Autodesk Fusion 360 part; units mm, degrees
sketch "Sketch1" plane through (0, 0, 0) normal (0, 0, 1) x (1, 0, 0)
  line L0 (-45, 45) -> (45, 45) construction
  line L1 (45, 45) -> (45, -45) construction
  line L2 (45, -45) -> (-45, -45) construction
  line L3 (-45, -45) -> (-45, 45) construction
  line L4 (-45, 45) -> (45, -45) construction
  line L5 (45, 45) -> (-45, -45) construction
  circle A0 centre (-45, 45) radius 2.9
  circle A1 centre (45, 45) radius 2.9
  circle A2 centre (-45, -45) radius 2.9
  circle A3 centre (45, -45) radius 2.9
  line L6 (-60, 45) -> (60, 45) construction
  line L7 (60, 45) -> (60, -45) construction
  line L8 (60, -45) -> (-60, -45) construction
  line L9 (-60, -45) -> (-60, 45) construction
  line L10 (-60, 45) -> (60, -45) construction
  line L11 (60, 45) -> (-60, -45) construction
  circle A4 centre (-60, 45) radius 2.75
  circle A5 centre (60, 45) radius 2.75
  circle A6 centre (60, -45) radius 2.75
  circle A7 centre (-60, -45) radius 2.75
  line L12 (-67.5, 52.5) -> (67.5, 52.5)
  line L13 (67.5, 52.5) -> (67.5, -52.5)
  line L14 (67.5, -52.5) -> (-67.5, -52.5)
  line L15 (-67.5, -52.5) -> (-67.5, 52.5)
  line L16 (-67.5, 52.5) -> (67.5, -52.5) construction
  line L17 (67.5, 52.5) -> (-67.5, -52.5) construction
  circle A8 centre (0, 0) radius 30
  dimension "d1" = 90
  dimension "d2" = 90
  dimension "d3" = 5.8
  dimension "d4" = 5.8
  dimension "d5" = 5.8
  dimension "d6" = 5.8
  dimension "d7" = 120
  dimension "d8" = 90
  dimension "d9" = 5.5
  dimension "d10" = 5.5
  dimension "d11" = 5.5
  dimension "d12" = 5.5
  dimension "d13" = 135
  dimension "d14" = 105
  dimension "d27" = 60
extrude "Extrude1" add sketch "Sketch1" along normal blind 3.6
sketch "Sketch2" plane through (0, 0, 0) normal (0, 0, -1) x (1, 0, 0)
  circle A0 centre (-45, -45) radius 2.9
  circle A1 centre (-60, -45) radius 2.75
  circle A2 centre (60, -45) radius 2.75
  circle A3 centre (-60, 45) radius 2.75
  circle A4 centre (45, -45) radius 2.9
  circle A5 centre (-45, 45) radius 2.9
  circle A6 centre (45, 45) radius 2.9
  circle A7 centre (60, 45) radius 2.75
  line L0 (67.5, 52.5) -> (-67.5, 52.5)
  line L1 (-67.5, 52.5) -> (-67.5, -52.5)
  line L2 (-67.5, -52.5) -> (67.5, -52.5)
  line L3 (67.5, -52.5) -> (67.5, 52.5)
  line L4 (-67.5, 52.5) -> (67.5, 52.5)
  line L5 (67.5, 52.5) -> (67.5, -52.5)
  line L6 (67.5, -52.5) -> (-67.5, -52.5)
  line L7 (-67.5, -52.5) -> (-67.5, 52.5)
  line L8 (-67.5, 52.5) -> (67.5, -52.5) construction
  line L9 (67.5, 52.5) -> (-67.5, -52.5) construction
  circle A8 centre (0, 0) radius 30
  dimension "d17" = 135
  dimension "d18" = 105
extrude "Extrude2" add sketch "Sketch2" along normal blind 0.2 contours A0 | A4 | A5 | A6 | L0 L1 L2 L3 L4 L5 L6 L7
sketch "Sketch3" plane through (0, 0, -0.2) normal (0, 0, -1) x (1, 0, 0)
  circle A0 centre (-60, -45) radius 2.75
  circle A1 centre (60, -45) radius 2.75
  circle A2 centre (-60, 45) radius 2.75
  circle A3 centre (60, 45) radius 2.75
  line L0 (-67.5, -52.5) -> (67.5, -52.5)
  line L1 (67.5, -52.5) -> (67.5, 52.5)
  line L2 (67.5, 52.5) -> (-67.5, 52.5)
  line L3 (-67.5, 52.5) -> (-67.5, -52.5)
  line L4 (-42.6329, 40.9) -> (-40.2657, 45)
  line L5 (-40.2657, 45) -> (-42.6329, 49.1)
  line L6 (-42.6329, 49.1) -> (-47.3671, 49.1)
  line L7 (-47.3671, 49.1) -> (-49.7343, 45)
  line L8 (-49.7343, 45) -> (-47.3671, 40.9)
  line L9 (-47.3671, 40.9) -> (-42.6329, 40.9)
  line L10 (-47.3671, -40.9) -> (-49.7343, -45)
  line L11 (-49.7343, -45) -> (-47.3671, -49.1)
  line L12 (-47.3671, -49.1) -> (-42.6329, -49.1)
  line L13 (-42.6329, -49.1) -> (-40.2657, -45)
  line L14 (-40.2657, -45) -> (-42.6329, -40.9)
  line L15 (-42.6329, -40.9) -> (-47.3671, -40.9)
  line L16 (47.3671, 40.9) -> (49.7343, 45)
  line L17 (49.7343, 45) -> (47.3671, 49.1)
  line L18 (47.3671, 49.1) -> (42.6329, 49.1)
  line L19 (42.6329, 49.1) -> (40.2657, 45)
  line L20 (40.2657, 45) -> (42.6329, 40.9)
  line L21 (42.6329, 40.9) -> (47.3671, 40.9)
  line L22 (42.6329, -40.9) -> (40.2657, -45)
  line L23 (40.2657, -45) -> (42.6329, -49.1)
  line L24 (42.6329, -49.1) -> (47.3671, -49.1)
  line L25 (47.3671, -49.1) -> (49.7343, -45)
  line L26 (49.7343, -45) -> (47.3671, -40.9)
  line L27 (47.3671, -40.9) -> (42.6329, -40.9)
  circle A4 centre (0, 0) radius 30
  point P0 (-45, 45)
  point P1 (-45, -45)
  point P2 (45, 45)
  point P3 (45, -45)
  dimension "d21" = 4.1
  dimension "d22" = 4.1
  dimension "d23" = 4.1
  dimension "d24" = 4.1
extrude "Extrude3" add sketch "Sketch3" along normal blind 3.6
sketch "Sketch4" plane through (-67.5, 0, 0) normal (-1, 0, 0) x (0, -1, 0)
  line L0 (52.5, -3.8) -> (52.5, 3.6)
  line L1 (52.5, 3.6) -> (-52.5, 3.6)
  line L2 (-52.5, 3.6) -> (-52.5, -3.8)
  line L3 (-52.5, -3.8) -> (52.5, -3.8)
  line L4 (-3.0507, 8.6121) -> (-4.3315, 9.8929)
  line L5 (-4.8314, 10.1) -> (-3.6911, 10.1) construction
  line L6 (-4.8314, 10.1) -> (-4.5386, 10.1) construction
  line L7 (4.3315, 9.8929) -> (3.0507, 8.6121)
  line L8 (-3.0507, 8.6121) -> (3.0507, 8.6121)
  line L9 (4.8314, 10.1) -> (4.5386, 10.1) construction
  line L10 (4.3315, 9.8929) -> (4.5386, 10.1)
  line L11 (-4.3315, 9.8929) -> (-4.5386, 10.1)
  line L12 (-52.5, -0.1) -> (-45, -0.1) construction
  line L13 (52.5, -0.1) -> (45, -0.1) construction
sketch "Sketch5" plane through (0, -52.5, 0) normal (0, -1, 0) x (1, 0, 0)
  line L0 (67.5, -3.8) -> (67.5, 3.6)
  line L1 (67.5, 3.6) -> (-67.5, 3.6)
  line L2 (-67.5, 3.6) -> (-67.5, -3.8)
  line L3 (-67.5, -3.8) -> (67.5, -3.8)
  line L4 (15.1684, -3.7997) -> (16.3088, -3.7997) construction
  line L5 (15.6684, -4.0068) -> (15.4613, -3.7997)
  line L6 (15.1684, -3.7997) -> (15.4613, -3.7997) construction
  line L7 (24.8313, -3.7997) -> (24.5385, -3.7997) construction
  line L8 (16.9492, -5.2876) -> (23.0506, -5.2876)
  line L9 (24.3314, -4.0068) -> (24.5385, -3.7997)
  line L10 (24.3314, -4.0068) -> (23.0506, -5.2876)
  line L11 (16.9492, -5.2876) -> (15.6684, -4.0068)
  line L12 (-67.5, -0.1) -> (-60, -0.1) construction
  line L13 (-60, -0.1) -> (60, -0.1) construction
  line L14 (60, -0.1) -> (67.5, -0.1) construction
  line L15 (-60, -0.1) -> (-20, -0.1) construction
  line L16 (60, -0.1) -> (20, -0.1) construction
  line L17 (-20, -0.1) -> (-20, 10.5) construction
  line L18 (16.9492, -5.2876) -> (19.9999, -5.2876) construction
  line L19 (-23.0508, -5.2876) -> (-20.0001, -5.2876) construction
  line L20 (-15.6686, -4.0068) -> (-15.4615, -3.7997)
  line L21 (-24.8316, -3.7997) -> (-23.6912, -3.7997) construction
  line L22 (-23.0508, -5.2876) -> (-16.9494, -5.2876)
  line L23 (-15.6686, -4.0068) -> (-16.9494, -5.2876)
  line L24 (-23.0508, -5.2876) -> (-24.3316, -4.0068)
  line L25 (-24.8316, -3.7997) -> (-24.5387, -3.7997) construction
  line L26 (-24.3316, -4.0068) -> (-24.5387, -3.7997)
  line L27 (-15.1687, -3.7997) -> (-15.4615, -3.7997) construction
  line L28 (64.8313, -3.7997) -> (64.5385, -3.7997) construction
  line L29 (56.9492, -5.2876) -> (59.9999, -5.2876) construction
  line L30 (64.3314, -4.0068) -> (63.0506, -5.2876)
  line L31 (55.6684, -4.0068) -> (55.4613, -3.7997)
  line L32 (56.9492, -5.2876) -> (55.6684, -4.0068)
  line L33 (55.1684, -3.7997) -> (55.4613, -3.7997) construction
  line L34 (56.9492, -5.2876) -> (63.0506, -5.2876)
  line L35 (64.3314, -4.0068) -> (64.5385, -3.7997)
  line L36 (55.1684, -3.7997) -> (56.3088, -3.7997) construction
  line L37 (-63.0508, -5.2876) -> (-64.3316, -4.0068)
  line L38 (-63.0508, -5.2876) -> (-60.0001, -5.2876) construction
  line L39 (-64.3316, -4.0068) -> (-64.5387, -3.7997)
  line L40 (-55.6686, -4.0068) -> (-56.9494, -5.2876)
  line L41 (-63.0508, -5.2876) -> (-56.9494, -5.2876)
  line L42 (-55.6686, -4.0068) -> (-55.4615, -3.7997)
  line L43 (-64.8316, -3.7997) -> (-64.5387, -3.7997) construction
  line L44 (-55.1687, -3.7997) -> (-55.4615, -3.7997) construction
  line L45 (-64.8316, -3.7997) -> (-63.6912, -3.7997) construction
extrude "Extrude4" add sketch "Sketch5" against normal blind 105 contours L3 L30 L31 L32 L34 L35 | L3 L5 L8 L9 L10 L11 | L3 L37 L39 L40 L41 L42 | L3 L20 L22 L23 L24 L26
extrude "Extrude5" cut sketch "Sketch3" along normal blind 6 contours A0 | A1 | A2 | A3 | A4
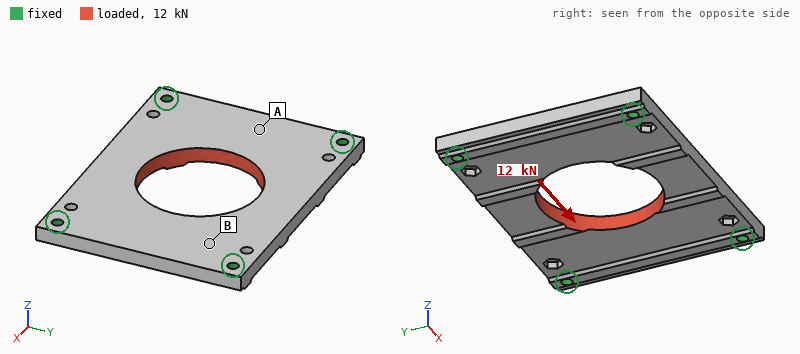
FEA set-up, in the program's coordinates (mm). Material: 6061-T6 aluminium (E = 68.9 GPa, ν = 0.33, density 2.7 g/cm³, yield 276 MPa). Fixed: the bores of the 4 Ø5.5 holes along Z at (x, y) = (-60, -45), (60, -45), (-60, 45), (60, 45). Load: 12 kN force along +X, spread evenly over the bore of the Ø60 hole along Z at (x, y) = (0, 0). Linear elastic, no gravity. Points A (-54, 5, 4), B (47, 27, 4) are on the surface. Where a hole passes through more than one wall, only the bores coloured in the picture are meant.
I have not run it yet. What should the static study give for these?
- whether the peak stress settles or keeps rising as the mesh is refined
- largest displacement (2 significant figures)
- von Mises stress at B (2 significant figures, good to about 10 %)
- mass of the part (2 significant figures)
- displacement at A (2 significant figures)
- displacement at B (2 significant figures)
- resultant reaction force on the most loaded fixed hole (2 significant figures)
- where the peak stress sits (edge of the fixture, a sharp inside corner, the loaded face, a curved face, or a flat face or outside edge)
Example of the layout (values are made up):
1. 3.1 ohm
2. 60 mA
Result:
1. keeps rising
2. 17 µm
3. 13 MPa
4. 230 g
5. 15 µm
6. 10 µm
7. 3.2 kN
8. edge of the fixture
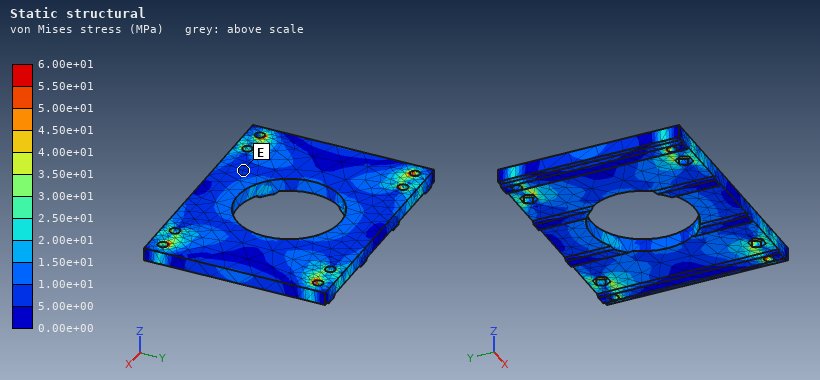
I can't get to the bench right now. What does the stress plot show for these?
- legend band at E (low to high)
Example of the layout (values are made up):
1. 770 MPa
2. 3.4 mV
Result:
1. 5.00e+00 to 1.00e+01 MPa
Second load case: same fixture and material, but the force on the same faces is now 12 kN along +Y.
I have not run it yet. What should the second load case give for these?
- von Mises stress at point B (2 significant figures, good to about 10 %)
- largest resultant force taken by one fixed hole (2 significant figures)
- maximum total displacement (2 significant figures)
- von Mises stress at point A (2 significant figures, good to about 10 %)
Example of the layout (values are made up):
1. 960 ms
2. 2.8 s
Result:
1. 15 MPa
2. 3.4 kN
3. 28 µm
4. 15 MPa
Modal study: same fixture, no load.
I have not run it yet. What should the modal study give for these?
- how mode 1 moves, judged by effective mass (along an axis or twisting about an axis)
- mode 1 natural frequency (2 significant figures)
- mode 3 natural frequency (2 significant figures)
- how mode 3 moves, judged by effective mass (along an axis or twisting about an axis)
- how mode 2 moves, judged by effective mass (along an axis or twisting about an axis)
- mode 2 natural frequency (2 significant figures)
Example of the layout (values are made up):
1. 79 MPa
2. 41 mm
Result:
1. along Z
2. 2300 Hz
3. 4200 Hz
4. twisting about Y
5. twisting about X
6. 3000 Hz
